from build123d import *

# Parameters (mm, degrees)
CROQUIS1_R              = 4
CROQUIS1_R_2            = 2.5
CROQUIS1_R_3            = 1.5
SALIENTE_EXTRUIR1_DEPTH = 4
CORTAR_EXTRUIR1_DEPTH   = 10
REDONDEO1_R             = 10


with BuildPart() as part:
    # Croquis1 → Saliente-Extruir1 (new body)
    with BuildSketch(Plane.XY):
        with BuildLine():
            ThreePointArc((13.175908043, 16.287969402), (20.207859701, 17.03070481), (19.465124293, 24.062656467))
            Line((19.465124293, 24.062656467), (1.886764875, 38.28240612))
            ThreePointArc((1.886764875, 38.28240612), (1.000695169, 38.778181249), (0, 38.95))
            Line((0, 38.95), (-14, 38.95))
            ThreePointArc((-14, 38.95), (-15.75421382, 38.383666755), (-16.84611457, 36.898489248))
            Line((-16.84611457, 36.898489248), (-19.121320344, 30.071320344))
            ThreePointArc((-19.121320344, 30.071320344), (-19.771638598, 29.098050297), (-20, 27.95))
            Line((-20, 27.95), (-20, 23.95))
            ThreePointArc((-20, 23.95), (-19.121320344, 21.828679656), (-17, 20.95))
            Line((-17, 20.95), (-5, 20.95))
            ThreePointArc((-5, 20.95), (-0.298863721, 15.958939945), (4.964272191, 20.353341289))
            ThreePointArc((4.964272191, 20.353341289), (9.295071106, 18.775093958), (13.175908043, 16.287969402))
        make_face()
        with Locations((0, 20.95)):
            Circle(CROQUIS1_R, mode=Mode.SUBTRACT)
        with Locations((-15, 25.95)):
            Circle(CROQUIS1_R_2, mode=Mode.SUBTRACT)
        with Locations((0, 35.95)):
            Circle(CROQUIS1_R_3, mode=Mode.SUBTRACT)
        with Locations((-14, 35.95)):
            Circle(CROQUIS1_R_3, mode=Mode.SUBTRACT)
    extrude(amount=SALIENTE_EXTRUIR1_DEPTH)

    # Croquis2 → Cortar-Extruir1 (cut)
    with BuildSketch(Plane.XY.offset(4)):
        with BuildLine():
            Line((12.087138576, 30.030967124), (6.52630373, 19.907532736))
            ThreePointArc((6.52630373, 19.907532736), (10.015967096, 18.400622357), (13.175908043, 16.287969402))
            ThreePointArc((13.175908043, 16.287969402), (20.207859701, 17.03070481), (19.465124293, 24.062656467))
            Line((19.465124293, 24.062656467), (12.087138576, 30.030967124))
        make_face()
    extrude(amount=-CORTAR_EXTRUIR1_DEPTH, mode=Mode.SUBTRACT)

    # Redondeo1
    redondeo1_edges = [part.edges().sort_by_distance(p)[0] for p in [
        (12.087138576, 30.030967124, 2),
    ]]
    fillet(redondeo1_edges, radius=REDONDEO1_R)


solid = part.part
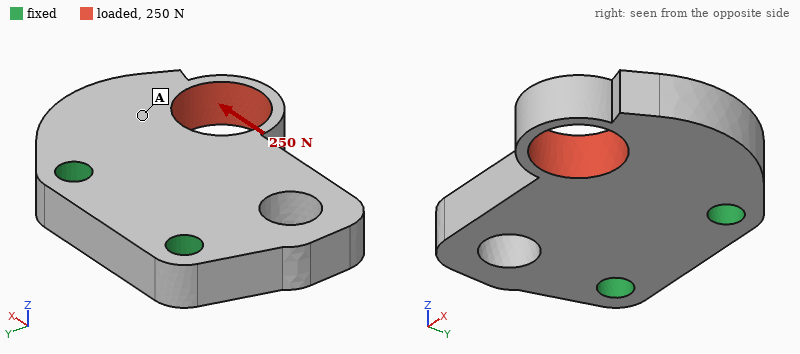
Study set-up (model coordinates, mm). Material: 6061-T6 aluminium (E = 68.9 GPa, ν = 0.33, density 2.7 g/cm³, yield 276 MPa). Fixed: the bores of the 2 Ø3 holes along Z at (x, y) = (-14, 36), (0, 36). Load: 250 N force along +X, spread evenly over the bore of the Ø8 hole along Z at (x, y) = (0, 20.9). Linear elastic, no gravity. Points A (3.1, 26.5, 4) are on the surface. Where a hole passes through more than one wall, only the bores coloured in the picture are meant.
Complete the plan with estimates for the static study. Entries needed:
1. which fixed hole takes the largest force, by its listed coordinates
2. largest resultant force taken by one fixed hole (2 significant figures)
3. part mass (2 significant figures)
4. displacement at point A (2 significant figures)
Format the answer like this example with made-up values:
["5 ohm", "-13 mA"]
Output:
["(-14, 36)", "280 N", "4.6 g", "3.0 µm"]
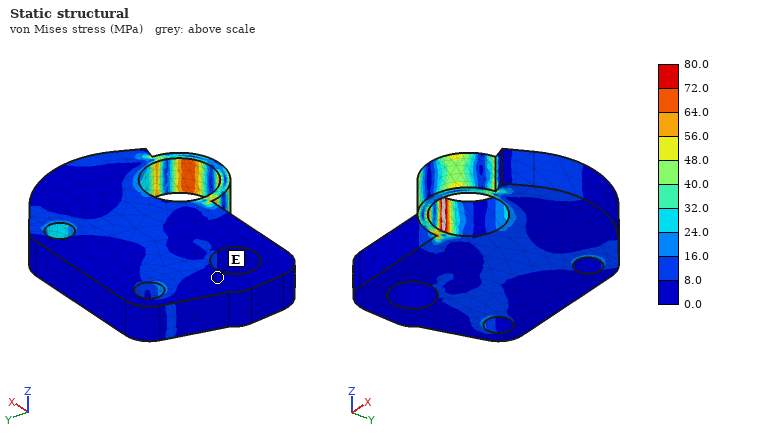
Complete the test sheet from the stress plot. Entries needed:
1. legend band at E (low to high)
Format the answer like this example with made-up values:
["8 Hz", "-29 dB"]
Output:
["0.0 to 8.0 MPa"]
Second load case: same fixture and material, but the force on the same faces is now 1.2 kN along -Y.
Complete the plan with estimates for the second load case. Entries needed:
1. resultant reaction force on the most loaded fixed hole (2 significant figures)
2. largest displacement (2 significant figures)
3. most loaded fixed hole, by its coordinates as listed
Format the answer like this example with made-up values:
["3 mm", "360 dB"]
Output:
["1.1 kN", "23 µm", "(0, 36)"]
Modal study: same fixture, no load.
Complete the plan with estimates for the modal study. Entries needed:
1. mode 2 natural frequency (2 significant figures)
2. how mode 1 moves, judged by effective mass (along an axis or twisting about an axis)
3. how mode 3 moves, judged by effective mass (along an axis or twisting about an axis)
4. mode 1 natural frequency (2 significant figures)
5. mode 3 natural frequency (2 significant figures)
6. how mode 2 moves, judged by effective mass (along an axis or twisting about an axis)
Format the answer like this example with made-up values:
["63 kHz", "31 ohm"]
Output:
["18 kHz", "along Z", "along X", "12 kHz", "29 kHz", "twisting about Y"]
